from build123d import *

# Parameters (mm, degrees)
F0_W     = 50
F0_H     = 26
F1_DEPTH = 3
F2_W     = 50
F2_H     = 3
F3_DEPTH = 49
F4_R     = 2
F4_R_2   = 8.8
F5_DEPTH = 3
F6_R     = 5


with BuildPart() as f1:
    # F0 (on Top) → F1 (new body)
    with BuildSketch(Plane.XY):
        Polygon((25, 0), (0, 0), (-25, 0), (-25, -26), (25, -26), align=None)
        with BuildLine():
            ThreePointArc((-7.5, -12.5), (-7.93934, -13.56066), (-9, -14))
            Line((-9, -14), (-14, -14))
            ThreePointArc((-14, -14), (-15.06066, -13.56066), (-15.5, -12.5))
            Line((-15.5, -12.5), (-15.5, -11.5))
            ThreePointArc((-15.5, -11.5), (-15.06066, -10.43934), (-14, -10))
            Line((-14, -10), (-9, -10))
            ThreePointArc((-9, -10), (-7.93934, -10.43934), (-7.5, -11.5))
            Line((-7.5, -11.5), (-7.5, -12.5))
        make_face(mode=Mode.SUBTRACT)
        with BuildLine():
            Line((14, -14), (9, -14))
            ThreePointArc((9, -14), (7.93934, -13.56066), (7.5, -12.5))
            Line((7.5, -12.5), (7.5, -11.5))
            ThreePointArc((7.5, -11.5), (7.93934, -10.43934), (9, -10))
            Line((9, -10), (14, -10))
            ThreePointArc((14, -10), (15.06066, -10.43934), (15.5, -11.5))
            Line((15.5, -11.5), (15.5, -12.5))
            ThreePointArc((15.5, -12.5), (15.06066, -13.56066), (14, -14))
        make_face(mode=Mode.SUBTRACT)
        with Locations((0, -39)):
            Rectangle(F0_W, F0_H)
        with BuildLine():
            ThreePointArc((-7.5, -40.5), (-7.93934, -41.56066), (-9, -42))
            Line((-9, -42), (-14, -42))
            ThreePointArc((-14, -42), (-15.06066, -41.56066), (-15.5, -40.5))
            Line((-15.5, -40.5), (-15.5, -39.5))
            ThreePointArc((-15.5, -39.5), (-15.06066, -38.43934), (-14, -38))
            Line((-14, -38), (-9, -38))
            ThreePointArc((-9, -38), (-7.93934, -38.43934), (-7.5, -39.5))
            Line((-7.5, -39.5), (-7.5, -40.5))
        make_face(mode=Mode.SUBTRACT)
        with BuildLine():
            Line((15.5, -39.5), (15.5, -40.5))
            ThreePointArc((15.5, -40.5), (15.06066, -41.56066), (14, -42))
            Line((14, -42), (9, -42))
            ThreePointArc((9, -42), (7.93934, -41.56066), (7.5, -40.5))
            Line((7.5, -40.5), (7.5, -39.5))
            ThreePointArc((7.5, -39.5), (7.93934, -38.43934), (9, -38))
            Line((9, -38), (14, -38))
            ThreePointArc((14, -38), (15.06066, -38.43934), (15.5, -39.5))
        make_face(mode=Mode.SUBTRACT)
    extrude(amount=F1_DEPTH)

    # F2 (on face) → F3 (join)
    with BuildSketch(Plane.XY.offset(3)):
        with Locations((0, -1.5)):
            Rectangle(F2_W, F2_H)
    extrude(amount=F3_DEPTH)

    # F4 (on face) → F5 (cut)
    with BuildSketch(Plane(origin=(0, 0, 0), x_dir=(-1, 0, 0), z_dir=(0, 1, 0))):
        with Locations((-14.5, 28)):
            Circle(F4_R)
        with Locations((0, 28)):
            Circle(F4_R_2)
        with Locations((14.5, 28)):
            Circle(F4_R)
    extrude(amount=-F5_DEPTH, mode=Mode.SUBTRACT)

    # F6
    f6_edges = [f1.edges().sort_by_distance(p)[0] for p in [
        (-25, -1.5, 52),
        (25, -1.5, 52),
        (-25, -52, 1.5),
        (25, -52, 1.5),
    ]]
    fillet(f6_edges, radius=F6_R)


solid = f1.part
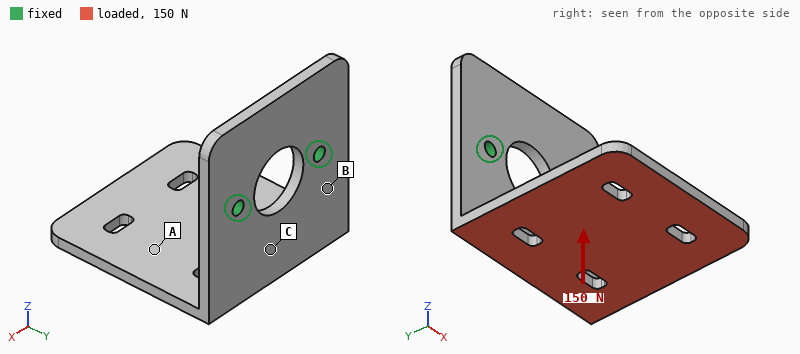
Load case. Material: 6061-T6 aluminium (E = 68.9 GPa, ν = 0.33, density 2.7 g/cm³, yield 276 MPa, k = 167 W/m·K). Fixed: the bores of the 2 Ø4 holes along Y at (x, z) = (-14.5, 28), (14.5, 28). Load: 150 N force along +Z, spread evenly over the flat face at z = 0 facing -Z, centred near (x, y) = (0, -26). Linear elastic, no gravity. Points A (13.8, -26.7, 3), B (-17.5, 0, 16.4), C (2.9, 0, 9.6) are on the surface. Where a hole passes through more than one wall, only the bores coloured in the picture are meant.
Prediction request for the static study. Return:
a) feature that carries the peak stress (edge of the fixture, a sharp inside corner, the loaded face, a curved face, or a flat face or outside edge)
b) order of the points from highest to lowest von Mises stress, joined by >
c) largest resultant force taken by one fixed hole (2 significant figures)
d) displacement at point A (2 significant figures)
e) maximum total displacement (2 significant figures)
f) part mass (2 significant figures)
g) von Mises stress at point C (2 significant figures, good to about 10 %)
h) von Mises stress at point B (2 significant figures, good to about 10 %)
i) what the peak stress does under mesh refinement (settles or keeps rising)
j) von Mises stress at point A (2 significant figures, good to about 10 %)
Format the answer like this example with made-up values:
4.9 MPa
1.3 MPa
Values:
edge of the fixture
B > C > A
79 N
0.48 mm
1.0 mm
38 g
39 MPa
51 MPa
keeps rising
11 MPa
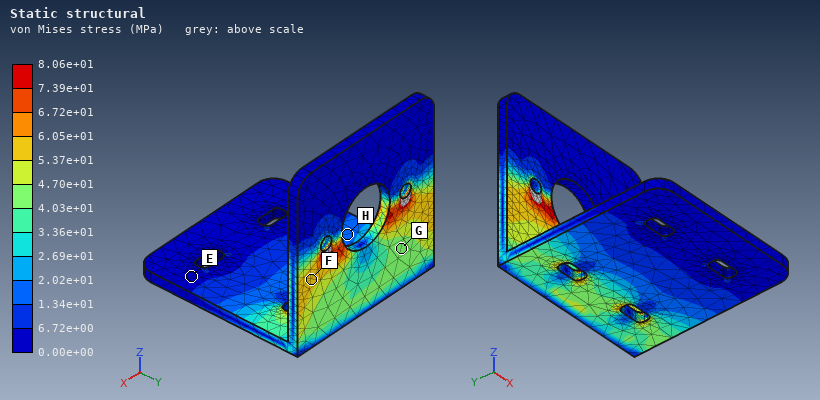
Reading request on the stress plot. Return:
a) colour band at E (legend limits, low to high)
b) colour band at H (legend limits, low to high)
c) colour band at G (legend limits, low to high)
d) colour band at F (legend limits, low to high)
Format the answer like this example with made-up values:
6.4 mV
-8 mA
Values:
0.00e+00 to 6.72e+00 MPa
1.34e+01 to 2.02e+01 MPa
4.03e+01 to 4.70e+01 MPa
5.37e+01 to 6.05e+01 MPa
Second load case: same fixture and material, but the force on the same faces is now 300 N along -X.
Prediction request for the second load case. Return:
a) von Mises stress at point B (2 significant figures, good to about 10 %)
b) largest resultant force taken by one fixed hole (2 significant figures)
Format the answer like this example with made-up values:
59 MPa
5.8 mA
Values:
40 MPa
350 N
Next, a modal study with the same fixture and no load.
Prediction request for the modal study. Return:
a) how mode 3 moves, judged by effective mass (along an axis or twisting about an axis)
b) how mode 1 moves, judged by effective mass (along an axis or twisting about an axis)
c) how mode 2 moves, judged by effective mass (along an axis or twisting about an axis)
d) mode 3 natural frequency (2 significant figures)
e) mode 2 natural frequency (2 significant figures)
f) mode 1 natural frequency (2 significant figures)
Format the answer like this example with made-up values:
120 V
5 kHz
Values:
along Y
along Z
along X
1700 Hz
1000 Hz
500 Hz
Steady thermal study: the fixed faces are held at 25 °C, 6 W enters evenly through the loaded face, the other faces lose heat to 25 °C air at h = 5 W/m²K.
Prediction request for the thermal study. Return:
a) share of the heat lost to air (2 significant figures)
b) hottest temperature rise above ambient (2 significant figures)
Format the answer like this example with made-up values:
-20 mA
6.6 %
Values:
4.0 %
14 K
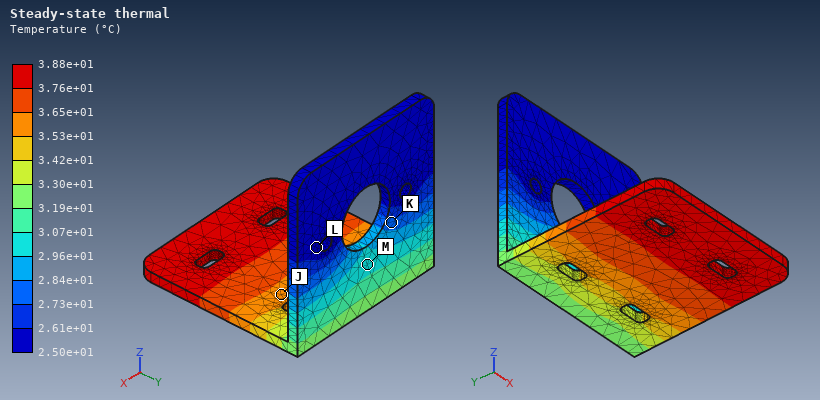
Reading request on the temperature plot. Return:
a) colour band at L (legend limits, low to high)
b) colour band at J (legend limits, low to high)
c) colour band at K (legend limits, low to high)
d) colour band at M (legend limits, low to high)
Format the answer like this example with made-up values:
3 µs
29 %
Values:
2.50e+01 to 2.61e+01 °C
3.53e+01 to 3.65e+01 °C
2.73e+01 to 2.84e+01 °C
2.96e+01 to 3.07e+01 °C
